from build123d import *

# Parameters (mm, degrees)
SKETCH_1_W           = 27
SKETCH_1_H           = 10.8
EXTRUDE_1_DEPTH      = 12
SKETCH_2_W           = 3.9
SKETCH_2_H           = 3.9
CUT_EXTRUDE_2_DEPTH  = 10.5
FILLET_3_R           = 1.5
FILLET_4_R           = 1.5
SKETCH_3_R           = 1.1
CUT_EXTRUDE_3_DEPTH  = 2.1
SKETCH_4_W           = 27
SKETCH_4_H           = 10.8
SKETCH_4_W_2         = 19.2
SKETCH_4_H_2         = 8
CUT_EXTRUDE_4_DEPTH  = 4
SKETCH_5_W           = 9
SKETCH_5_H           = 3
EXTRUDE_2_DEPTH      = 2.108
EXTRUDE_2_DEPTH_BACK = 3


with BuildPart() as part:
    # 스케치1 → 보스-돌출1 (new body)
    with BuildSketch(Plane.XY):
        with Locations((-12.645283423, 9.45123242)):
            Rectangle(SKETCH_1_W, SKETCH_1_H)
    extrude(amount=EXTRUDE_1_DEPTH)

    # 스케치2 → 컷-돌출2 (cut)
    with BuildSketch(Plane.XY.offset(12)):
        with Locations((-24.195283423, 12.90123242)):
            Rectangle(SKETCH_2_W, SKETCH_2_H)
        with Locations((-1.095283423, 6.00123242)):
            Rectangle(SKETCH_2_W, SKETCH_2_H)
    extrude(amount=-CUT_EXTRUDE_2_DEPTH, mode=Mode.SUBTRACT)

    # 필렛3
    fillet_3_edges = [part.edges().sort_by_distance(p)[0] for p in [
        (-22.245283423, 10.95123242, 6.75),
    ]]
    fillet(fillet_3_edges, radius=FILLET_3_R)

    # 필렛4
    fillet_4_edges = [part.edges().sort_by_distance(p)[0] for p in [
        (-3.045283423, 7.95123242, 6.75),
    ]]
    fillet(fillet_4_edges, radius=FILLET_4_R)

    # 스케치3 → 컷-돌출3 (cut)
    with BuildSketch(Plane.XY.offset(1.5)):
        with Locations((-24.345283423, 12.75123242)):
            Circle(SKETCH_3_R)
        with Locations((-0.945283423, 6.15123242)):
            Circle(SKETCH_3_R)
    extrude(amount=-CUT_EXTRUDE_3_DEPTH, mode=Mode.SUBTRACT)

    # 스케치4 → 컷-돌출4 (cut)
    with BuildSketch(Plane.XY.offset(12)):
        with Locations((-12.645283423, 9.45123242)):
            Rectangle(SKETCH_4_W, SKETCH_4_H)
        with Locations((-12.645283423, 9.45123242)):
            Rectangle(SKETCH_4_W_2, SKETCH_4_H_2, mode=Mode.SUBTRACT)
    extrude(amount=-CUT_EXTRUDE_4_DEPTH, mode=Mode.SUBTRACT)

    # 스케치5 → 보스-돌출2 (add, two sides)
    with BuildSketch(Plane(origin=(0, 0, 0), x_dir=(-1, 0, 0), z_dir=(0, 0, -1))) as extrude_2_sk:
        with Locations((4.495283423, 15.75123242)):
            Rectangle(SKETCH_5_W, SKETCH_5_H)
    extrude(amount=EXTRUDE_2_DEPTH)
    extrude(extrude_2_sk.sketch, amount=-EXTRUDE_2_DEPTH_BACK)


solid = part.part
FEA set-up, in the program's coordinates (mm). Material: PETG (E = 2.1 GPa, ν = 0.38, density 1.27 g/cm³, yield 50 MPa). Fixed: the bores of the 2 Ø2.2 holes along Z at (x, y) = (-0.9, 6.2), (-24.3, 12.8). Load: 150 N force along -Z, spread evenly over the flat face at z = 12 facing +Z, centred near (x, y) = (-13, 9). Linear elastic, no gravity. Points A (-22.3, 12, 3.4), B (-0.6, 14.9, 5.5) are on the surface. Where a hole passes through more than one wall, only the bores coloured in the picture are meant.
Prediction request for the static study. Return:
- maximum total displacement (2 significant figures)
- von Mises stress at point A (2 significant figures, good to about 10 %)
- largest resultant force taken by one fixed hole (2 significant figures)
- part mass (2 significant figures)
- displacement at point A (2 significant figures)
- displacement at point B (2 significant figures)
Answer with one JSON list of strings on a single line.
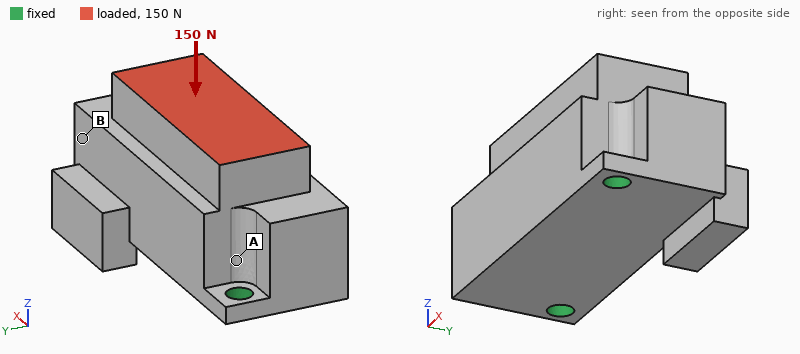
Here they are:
["49 µm", "4.7 MPa", "84 N", "3.6 g", "32 µm", "41 µm"]
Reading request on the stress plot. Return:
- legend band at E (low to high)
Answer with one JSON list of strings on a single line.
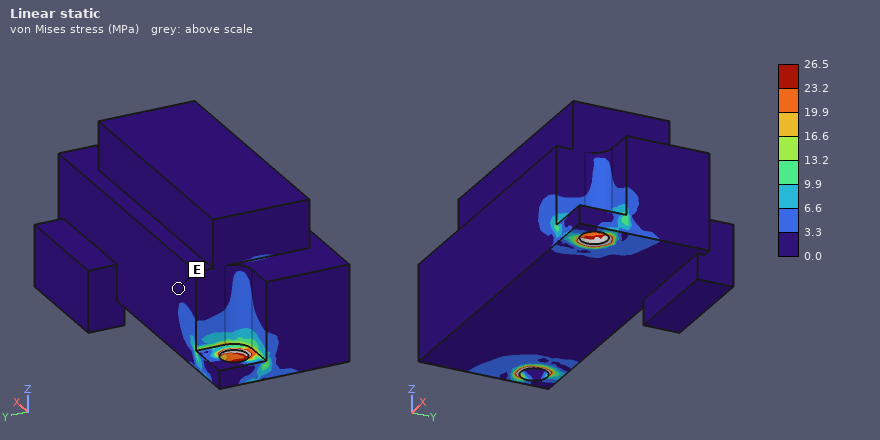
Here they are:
["0.0 to 3.3 MPa"]
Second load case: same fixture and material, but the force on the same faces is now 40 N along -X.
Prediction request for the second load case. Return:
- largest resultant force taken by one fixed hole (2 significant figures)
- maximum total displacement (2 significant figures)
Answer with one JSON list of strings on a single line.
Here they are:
["27 N", "0.13 mm"]
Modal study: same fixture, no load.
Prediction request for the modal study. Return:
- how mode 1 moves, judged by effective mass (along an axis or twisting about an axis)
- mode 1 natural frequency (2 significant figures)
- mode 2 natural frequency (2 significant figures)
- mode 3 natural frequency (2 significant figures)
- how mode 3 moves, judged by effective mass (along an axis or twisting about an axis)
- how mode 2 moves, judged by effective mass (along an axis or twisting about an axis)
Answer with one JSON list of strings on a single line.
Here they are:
["along Y", "1300 Hz", "5000 Hz", "6500 Hz", "along X", "along Z"]
